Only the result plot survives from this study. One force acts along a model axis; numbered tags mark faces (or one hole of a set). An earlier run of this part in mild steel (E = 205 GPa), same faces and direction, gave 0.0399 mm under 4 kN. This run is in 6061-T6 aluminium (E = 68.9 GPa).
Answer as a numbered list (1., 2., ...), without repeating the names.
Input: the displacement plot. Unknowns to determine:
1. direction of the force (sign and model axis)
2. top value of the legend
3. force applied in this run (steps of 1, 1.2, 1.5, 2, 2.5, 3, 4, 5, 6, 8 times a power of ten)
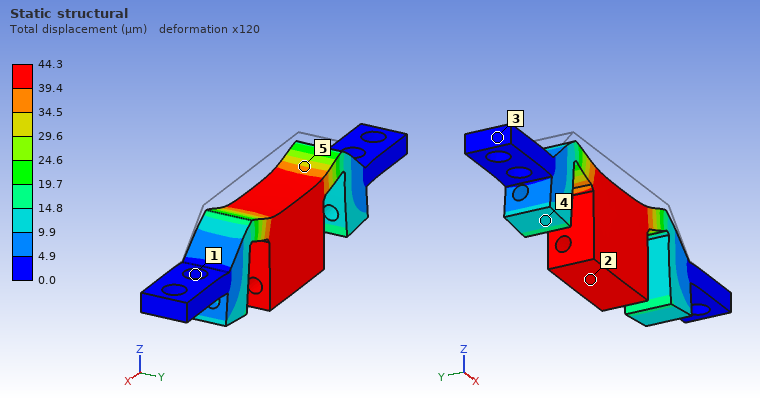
1. -Z
2. 44.3 µm
3. 1.5 kN
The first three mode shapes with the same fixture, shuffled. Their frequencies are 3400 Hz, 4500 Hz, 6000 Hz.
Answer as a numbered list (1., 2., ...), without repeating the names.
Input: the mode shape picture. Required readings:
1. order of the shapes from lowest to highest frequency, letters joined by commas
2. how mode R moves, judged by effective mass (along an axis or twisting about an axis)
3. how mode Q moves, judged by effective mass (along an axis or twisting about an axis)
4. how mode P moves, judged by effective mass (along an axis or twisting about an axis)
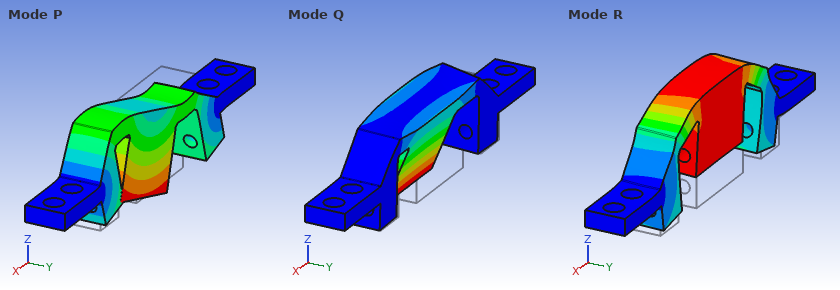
1. Q, P, R
2. along Z
3. along Y
4. along X
